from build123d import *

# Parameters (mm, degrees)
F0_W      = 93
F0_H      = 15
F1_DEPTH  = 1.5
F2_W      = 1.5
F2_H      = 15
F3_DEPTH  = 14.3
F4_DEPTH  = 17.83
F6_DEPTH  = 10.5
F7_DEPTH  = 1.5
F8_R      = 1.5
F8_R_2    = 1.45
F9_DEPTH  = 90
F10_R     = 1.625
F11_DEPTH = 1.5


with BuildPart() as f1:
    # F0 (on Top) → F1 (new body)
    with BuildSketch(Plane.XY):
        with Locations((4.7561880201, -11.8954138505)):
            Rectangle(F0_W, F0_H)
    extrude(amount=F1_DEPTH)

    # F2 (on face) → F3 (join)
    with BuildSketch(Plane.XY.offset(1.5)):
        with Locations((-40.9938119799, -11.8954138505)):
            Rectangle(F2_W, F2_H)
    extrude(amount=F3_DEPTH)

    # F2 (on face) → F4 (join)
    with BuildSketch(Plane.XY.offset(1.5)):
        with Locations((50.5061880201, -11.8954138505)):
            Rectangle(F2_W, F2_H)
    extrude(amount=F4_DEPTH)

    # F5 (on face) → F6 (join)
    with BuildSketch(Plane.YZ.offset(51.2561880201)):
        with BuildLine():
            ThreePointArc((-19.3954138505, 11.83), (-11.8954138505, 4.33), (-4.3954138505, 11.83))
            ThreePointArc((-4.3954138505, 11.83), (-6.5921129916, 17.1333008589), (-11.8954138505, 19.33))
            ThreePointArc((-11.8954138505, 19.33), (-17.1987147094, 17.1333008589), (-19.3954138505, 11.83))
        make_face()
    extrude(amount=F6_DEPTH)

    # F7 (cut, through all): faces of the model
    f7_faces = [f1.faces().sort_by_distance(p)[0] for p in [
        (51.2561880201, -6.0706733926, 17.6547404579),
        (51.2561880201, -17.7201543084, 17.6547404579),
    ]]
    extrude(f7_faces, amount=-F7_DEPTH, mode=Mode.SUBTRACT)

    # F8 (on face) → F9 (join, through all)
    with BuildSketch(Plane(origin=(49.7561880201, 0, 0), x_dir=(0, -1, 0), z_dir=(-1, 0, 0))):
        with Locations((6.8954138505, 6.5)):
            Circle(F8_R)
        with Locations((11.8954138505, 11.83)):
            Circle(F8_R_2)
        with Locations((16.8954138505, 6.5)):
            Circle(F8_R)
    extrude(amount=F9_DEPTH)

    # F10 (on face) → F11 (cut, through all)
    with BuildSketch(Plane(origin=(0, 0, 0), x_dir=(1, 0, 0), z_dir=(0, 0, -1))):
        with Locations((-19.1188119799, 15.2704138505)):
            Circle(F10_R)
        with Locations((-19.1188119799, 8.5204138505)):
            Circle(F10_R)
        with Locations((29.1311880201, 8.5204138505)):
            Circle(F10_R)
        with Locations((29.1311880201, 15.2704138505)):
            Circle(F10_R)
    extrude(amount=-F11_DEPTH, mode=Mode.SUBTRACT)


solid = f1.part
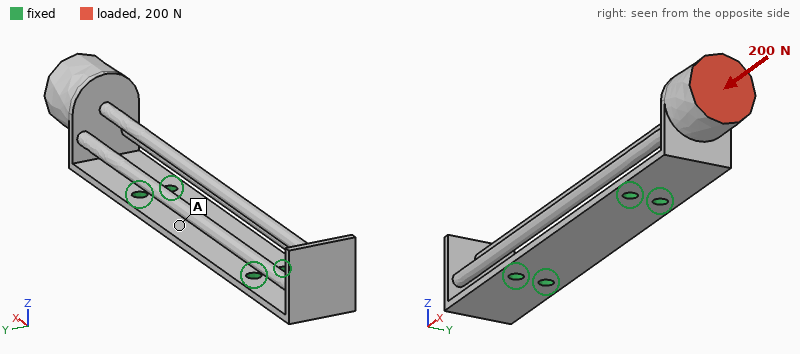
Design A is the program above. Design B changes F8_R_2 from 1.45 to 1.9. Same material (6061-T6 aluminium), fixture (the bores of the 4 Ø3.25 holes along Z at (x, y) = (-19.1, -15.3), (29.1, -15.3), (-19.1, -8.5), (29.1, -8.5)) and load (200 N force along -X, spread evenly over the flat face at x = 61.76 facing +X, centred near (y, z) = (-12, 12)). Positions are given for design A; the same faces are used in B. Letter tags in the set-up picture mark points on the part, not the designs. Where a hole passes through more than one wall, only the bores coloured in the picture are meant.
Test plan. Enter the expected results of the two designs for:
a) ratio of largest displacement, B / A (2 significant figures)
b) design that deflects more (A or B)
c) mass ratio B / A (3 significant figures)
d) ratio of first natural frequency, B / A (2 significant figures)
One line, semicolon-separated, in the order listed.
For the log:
0.80; A; 1.07; 1.0
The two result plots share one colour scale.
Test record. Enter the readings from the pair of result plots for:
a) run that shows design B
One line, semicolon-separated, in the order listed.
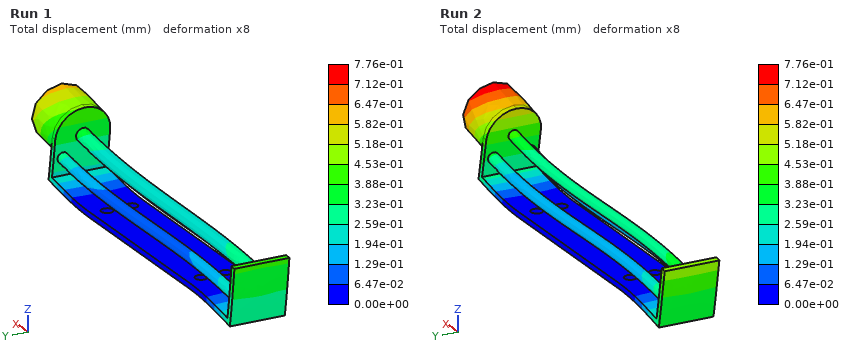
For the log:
Run 1
